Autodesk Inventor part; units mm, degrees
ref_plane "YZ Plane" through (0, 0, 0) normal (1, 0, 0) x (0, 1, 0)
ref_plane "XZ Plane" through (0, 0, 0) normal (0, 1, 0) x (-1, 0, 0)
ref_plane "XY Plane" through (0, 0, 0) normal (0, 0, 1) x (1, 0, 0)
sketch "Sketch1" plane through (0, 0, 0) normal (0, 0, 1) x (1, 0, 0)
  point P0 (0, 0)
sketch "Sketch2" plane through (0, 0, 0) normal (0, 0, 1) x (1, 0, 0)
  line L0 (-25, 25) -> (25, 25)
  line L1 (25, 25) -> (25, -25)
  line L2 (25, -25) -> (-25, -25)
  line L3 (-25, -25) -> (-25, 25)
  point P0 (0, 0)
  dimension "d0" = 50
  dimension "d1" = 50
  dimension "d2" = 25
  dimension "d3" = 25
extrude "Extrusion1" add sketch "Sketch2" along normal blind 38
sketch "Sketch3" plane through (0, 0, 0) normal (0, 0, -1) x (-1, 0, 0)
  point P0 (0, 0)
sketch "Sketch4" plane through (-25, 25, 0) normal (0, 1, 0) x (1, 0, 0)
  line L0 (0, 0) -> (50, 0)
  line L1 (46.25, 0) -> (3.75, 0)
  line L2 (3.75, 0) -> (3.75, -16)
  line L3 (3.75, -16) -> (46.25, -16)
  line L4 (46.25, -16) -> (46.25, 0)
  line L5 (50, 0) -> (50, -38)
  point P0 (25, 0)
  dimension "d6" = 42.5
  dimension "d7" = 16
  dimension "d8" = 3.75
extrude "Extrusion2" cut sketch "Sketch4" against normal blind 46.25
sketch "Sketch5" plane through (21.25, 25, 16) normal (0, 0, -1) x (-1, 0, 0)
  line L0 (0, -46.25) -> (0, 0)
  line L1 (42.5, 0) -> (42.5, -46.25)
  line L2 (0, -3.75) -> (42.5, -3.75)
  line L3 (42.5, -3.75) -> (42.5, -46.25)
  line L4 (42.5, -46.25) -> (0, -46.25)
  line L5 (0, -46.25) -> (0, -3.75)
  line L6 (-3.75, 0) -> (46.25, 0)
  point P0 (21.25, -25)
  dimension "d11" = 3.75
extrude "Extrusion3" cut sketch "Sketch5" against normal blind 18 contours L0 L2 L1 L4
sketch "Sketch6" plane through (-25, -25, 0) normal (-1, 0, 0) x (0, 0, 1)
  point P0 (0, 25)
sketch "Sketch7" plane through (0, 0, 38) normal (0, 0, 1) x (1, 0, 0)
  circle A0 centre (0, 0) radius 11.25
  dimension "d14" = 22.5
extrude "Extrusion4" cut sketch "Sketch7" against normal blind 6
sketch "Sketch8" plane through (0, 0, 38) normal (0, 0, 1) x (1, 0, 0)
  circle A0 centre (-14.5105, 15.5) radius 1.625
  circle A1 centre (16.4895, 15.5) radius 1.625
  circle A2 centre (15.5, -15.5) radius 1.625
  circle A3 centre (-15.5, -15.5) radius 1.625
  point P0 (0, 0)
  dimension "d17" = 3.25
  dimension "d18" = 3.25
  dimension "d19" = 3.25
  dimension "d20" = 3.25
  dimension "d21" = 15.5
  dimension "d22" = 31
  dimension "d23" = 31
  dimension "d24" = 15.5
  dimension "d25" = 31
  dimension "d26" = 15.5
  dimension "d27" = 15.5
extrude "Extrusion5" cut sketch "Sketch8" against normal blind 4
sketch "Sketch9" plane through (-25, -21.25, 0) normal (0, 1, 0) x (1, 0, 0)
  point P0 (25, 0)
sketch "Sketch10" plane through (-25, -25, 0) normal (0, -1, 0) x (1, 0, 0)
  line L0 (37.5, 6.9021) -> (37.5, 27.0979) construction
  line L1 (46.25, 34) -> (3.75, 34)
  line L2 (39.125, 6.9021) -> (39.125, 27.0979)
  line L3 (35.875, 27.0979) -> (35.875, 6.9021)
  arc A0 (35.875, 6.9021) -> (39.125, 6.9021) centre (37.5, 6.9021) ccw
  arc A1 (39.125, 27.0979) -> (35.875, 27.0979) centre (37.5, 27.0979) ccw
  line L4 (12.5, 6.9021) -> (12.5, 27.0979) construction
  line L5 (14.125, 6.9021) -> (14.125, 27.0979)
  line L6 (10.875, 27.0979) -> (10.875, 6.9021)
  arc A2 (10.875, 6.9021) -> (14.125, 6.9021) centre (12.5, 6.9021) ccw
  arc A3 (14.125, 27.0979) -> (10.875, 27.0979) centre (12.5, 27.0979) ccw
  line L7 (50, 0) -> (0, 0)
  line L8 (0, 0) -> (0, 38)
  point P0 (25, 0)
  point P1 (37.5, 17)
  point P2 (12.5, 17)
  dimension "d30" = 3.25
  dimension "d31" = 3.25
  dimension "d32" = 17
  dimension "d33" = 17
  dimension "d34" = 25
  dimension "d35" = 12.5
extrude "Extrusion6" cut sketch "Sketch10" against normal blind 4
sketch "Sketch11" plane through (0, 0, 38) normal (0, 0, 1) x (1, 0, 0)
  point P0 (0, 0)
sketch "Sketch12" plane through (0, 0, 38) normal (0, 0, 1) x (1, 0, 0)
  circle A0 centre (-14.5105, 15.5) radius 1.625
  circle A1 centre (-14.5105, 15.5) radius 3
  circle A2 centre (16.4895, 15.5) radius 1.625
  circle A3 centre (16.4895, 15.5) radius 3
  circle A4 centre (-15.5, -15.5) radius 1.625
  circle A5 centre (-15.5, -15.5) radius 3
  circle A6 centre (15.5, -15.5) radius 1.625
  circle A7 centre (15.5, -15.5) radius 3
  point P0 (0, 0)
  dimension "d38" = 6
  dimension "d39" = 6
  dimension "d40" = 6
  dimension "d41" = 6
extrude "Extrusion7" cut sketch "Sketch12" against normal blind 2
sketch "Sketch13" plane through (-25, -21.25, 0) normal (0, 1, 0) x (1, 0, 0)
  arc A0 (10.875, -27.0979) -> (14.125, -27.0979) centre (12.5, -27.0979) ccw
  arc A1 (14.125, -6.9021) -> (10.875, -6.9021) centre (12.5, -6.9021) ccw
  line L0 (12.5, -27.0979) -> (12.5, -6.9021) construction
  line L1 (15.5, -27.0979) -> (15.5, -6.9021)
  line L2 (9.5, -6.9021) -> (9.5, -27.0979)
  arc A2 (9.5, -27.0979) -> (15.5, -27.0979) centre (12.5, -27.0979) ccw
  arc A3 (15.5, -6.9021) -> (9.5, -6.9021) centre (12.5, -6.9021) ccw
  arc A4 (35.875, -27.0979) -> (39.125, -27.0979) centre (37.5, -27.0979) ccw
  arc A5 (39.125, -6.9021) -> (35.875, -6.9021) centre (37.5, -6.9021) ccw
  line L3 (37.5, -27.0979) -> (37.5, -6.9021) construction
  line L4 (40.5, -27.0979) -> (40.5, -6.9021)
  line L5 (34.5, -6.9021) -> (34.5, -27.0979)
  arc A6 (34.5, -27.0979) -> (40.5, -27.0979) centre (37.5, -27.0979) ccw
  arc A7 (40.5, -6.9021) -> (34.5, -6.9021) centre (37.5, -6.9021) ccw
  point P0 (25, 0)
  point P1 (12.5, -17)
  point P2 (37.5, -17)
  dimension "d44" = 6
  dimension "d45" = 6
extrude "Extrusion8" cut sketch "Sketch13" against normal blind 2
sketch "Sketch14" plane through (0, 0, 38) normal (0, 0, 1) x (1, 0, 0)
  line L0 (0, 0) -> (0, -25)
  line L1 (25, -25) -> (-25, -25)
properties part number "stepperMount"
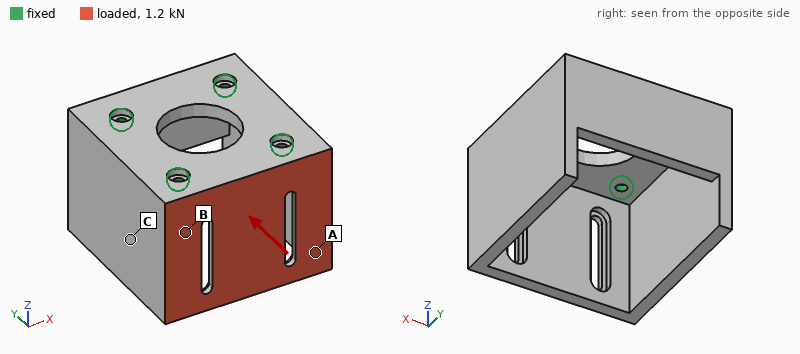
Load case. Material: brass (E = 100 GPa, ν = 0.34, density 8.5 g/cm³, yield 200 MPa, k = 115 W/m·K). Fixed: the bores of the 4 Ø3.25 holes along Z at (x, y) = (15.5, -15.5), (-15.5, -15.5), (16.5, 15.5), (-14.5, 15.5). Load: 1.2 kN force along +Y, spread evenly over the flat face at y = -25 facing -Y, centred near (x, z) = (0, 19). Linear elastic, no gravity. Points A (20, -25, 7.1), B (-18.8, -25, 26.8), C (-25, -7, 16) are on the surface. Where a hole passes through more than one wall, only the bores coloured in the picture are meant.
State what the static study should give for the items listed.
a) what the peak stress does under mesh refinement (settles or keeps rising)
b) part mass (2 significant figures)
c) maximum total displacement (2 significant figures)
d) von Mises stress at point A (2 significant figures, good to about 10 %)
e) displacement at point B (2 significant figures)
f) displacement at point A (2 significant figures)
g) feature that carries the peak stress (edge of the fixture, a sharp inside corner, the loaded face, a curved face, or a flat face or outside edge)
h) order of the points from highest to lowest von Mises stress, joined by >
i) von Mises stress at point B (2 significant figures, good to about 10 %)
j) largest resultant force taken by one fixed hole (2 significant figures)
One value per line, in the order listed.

keeps rising
240 g
55 µm
25 MPa
9.6 µm
16 µm
edge of the fixture
A > B > C
14 MPa
540 N
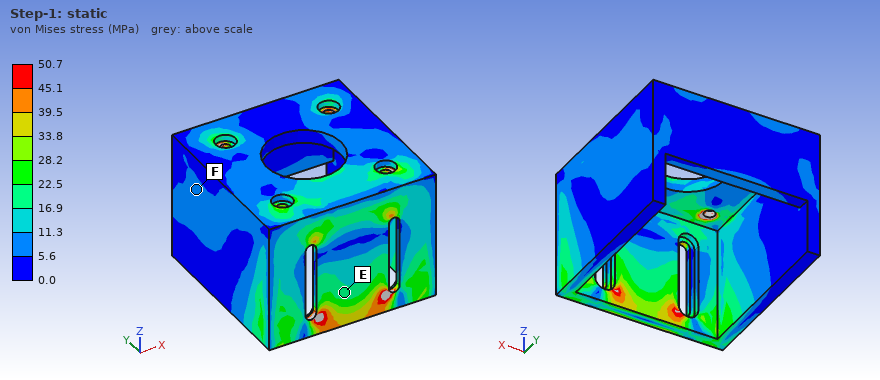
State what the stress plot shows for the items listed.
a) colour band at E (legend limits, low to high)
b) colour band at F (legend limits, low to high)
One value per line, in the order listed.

16.9 to 22.5 MPa
5.6 to 11.3 MPa
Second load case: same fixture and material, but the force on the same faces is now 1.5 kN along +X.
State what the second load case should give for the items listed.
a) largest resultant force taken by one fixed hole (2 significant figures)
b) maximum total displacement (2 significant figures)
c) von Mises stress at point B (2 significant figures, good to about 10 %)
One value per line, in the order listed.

1.1 kN
37 µm
19 MPa
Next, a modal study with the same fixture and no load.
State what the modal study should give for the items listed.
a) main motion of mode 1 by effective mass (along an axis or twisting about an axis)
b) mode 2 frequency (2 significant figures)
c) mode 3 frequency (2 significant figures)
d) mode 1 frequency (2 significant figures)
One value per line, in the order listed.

along X
3200 Hz
3500 Hz
3000 Hz
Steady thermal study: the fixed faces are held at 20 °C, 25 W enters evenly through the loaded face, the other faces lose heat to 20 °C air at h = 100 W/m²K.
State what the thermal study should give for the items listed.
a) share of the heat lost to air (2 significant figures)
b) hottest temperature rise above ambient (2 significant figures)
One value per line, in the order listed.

32 %
19 K
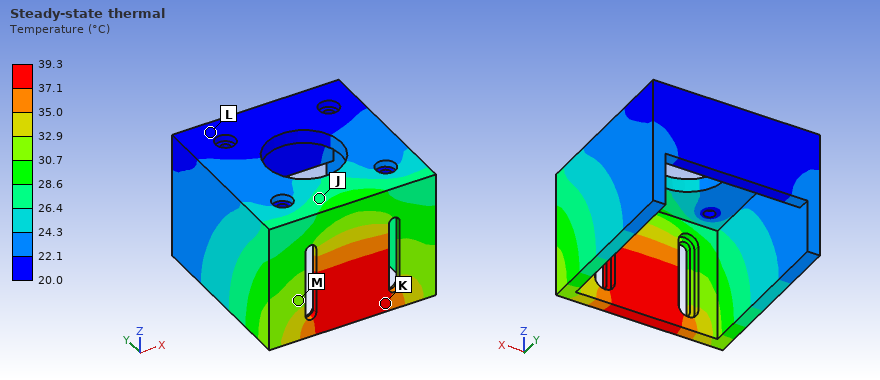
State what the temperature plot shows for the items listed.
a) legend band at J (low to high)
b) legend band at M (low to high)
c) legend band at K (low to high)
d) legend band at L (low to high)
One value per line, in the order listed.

26.4 to 28.6 °C
30.7 to 32.9 °C
37.1 to 39.3 °C
20.0 to 22.1 °C
